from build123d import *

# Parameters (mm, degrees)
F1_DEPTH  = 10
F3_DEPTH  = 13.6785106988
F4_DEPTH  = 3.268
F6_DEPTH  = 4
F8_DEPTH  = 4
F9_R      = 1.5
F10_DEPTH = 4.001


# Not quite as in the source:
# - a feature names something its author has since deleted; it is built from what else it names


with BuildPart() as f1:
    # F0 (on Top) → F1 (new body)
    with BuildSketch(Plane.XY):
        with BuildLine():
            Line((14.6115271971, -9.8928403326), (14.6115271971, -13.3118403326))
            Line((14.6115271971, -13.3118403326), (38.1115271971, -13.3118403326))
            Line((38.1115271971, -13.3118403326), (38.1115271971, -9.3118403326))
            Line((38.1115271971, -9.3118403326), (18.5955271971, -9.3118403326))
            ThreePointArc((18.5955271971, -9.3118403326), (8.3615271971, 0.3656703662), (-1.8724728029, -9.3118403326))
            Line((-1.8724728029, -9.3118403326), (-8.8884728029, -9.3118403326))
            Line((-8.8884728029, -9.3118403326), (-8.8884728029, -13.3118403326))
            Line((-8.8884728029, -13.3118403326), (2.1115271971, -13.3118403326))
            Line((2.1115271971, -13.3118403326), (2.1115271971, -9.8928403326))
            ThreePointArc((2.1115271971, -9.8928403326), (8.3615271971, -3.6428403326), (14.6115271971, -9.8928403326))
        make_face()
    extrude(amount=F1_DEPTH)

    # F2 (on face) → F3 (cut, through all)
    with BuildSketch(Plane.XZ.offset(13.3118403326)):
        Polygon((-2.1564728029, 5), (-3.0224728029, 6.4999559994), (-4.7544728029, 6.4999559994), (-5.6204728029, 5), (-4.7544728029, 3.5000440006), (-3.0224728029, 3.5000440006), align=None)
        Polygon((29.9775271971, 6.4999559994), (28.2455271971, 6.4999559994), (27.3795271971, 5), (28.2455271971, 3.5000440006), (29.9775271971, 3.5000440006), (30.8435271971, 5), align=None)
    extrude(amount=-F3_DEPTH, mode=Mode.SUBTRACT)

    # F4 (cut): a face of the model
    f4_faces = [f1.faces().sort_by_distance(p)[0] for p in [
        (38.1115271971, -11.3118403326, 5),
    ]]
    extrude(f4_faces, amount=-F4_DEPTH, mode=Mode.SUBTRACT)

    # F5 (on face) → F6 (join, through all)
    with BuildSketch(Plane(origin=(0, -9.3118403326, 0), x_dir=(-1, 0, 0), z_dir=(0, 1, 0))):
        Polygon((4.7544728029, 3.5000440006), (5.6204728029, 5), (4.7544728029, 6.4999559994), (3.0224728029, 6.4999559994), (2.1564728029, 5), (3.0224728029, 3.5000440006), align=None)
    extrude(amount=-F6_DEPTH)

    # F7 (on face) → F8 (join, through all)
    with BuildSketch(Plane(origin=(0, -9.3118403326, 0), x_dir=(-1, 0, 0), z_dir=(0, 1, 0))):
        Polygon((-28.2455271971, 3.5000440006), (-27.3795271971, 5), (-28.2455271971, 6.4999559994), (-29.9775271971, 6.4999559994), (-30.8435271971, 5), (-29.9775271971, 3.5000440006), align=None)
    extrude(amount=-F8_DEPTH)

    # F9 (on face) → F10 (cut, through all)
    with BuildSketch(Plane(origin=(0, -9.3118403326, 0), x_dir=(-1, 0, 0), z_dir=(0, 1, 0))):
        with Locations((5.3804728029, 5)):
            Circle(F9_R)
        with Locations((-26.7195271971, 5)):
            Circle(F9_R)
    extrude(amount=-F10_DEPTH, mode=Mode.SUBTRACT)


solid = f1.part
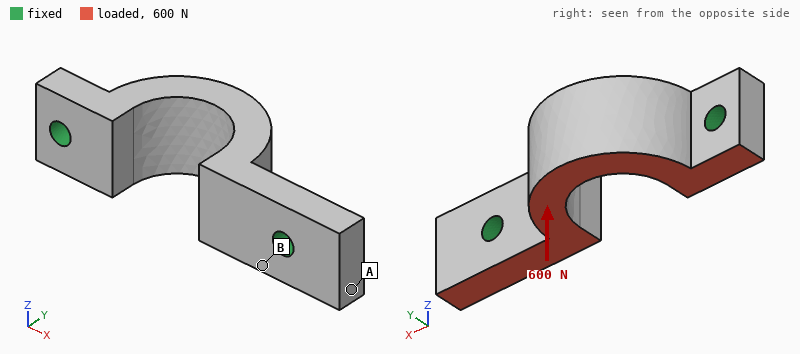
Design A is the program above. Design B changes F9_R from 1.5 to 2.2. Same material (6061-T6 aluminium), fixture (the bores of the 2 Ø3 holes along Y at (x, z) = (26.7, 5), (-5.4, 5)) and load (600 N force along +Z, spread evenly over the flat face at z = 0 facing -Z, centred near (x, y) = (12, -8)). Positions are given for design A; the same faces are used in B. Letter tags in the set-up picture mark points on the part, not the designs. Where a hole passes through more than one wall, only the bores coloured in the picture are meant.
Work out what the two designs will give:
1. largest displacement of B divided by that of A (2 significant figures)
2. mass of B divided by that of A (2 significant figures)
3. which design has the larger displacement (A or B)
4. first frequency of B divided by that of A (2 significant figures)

0.75
0.97
A
1.2
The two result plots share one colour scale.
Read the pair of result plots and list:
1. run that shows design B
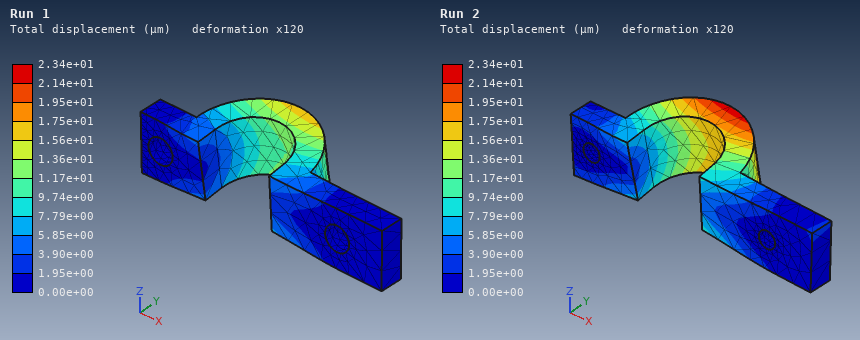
Run 1
